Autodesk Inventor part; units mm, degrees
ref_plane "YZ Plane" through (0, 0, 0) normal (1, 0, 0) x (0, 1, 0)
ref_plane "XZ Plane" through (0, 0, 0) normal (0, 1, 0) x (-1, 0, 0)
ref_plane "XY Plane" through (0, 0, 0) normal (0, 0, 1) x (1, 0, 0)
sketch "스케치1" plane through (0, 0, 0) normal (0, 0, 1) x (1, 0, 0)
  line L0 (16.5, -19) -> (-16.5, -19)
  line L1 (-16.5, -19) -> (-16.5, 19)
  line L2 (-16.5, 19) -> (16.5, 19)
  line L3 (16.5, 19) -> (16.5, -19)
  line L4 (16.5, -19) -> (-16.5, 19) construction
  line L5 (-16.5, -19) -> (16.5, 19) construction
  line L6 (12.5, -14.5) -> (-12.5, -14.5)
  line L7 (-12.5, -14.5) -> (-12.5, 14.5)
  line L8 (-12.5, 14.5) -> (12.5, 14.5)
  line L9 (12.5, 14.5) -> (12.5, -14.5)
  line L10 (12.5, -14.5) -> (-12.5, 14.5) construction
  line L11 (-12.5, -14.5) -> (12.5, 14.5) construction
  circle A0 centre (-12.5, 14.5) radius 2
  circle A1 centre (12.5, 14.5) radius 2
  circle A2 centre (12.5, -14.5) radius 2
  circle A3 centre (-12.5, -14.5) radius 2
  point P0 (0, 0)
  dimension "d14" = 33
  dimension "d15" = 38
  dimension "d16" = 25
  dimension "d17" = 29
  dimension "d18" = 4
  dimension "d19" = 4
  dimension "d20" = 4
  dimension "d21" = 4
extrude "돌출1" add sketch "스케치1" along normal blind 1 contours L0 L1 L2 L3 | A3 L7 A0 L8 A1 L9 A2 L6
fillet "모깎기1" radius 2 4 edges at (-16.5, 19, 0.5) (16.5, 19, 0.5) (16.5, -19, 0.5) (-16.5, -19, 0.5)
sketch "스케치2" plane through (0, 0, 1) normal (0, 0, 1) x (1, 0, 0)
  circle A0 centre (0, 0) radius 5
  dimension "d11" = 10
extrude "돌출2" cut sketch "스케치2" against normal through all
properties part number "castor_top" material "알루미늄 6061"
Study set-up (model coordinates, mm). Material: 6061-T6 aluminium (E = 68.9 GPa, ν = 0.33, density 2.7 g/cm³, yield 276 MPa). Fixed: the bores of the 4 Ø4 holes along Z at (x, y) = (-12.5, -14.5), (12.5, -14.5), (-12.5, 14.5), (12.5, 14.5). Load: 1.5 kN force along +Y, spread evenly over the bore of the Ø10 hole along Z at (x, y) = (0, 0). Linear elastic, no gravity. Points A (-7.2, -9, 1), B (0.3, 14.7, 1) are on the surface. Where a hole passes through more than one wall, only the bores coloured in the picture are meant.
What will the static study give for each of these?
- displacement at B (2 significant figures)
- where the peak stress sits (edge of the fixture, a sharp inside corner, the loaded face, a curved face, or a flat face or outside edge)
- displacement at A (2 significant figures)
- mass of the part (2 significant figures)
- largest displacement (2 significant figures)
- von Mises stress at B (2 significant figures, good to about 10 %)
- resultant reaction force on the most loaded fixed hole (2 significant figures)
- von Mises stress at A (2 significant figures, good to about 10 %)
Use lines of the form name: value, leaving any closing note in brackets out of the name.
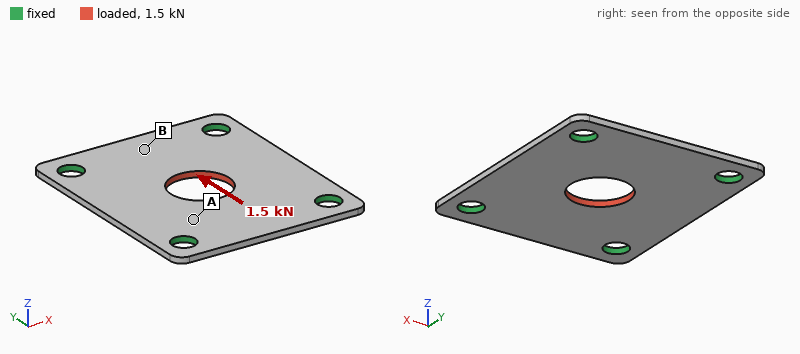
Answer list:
displacement at B: 7.7 µm
where the peak stress sits: edge of the fixture
displacement at A: 5.3 µm
mass of the part: 3.0 g
largest displacement: 11 µm
von Mises stress at B: 10 MPa
resultant reaction force on the most loaded fixed hole: 410 N
von Mises stress at A: 44 MPa
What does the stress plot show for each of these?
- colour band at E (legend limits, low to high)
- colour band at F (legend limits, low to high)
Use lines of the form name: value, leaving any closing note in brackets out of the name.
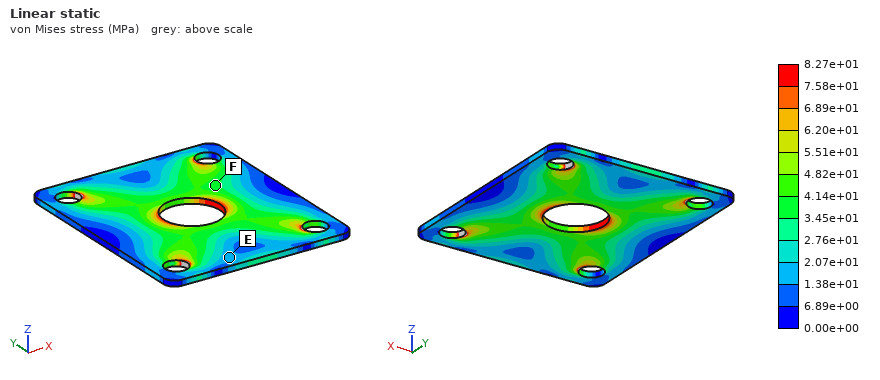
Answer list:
colour band at E: 1.38e+01 to 2.07e+01 MPa
colour band at F: 3.45e+01 to 4.14e+01 MPa
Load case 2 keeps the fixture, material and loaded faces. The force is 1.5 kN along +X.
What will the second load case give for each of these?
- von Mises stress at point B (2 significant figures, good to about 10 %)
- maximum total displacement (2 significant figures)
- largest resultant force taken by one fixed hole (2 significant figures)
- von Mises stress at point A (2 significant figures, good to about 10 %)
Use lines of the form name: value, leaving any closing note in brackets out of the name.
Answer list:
von Mises stress at point B: 16 MPa
maximum total displacement: 15 µm
largest resultant force taken by one fixed hole: 430 N
von Mises stress at point A: 48 MPa
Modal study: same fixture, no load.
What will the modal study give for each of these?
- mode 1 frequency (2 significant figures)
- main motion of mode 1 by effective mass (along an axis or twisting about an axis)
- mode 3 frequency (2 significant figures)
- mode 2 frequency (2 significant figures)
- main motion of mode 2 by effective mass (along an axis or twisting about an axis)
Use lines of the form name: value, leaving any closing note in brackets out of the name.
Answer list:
mode 1 frequency: 6200 Hz
main motion of mode 1 by effective mass: along Z
mode 3 frequency: 9800 Hz
mode 2 frequency: 8400 Hz
main motion of mode 2 by effective mass: twisting about Y
